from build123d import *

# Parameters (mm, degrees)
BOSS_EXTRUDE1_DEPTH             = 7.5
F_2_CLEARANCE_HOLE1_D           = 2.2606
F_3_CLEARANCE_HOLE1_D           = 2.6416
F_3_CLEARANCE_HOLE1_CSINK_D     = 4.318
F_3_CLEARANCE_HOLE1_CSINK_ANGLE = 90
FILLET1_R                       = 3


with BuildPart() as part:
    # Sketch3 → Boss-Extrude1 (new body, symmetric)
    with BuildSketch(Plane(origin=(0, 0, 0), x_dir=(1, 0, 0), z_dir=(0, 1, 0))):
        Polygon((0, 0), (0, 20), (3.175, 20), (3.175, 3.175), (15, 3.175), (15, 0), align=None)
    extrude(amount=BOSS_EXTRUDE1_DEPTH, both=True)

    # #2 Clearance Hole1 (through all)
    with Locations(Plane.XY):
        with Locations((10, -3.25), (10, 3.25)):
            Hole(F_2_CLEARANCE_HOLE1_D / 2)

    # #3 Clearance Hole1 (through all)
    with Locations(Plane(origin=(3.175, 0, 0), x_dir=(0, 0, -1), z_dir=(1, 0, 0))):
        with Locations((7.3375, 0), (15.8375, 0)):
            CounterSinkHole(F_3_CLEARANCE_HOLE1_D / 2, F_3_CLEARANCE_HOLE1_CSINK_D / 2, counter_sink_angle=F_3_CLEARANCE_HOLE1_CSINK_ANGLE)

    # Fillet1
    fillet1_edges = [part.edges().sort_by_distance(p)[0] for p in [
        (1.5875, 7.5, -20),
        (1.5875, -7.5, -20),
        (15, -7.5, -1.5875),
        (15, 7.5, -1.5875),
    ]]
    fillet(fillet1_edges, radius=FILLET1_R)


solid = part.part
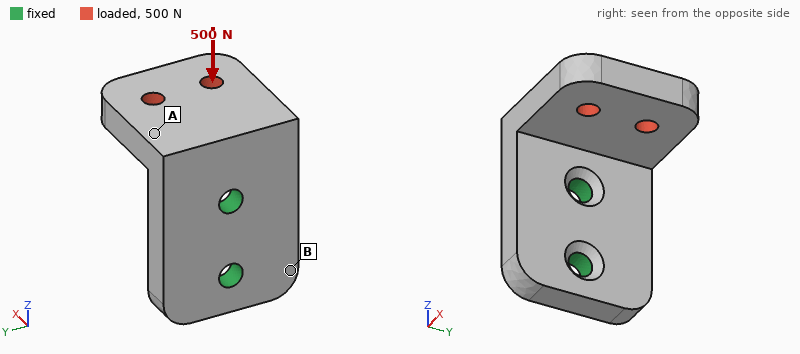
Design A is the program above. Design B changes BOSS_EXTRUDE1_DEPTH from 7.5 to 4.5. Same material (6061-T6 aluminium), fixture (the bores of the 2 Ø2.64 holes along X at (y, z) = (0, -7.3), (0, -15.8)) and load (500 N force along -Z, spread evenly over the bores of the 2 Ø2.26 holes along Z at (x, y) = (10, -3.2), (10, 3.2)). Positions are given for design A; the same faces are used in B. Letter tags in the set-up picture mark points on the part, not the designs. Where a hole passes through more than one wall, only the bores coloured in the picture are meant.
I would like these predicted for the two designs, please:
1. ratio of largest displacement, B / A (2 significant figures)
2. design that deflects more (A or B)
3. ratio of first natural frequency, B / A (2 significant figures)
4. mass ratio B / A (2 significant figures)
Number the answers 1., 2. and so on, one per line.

1. 1.6
2. B
3. 1.1
4. 0.57
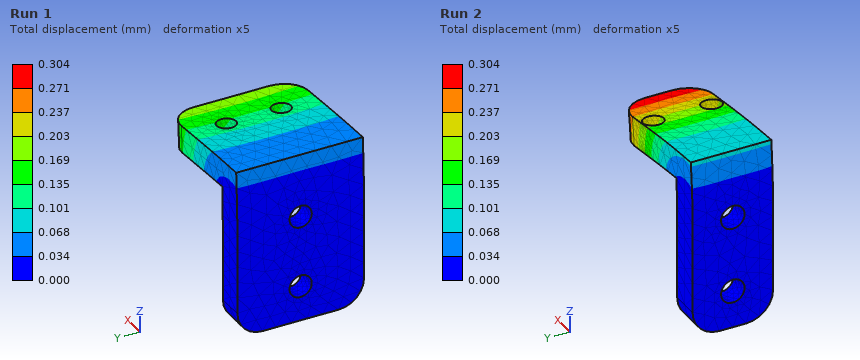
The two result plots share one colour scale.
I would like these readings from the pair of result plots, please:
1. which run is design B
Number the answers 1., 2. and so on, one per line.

1. Run 2
